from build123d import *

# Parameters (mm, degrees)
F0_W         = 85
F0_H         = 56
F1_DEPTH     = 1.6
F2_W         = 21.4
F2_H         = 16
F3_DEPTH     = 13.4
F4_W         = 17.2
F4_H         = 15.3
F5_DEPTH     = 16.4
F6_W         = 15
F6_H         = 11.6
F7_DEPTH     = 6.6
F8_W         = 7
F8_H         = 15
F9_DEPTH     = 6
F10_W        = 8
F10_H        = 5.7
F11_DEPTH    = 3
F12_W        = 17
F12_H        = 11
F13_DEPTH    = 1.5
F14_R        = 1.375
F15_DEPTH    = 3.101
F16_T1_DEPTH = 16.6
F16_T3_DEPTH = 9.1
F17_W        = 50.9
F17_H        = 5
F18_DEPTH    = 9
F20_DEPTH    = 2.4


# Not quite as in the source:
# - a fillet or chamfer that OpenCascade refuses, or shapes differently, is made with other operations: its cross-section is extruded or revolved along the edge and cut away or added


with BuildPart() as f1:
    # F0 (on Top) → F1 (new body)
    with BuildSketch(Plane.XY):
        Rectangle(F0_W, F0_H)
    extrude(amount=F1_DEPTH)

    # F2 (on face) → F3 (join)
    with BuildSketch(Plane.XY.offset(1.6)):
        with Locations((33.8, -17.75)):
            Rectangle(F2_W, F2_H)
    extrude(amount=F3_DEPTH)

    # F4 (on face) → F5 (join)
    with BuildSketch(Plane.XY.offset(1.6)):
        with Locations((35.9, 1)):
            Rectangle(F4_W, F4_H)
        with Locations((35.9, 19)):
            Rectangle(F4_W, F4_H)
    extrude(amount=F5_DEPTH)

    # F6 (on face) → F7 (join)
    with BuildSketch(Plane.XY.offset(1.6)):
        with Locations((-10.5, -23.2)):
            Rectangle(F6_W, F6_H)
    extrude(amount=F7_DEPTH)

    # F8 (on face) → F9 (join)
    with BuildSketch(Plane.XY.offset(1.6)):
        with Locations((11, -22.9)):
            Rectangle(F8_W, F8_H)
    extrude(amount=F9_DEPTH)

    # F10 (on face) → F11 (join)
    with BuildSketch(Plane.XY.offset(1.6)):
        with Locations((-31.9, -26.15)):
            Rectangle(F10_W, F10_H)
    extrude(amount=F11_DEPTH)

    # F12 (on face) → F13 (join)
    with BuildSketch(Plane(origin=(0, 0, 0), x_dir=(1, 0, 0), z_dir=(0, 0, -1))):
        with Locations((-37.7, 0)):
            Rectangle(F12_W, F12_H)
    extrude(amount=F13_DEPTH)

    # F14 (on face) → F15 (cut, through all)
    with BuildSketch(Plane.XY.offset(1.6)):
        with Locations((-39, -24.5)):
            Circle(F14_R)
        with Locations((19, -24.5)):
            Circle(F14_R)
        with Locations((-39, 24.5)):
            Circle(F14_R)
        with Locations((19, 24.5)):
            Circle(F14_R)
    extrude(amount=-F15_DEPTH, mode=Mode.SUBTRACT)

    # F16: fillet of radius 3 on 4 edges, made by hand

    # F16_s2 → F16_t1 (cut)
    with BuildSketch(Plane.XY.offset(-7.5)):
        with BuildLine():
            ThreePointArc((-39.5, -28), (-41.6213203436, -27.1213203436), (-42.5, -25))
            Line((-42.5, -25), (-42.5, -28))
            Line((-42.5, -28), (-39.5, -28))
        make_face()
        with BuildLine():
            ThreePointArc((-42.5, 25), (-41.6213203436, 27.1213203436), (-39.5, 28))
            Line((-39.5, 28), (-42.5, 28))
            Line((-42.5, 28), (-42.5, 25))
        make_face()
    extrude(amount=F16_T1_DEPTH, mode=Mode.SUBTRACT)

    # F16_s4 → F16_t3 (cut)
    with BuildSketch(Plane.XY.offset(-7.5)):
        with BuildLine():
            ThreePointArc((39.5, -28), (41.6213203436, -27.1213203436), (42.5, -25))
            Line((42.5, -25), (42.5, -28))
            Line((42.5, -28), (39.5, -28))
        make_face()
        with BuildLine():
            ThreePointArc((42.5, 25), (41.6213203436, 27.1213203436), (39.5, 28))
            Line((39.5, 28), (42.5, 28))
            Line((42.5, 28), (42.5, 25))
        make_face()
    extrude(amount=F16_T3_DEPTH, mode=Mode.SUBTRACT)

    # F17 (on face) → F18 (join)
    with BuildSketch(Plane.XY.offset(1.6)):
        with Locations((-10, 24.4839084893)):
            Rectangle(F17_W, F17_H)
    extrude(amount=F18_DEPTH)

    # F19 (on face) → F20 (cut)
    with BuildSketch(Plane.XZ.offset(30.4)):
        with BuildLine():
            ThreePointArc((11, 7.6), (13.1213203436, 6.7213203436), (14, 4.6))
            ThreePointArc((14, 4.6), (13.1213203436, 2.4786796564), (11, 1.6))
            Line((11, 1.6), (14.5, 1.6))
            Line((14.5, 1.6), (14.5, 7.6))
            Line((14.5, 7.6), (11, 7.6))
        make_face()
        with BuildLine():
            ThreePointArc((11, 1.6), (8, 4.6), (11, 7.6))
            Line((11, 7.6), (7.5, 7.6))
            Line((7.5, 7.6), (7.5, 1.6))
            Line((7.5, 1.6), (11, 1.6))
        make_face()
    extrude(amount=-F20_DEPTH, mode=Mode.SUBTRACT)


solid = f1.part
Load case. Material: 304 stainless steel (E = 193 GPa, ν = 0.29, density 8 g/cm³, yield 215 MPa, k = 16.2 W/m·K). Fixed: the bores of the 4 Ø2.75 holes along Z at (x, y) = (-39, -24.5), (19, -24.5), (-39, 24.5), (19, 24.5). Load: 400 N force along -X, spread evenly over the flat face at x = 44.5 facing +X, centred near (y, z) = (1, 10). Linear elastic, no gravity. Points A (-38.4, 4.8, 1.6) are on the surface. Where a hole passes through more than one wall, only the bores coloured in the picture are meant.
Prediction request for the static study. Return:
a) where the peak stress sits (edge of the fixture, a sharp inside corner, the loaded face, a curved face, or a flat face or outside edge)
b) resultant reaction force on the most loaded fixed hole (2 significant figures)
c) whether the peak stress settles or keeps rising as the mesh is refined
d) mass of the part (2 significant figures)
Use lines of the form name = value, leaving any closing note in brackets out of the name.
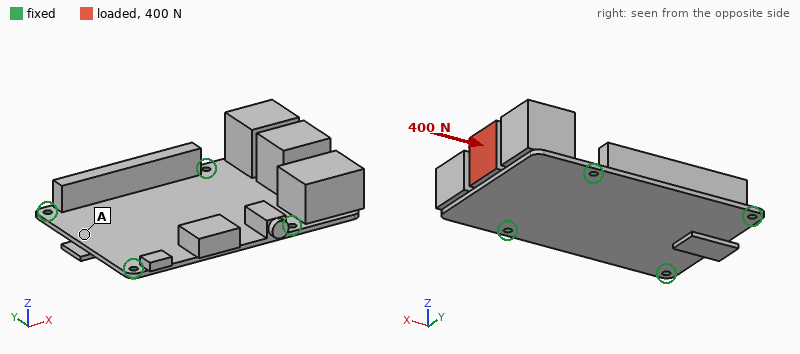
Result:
where the peak stress sits = edge of the fixture
resultant reaction force on the most loaded fixed hole = 150 N
whether the peak stress settles or keeps rising as the mesh is refined = keeps rising
mass of the part = 200 g
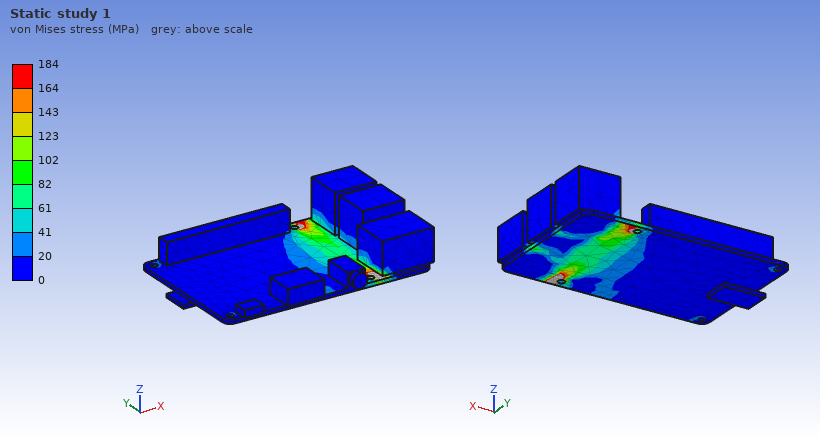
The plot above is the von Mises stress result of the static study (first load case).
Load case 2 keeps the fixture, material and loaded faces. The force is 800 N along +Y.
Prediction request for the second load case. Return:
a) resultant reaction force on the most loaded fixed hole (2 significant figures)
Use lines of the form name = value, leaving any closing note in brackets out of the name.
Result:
resultant reaction force on the most loaded fixed hole = 590 N
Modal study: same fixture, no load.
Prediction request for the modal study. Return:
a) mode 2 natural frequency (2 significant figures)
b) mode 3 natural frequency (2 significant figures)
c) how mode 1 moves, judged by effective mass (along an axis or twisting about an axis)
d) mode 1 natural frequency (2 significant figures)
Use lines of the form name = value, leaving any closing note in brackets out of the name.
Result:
mode 2 natural frequency = 1700 Hz
mode 3 natural frequency = 2000 Hz
how mode 1 moves, judged by effective mass = along Z
mode 1 natural frequency = 530 Hz
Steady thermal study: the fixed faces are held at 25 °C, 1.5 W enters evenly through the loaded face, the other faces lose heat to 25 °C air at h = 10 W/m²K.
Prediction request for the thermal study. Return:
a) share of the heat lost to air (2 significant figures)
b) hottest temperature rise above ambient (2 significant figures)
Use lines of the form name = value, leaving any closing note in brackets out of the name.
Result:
share of the heat lost to air = 51 %
hottest temperature rise above ambient = 20 K
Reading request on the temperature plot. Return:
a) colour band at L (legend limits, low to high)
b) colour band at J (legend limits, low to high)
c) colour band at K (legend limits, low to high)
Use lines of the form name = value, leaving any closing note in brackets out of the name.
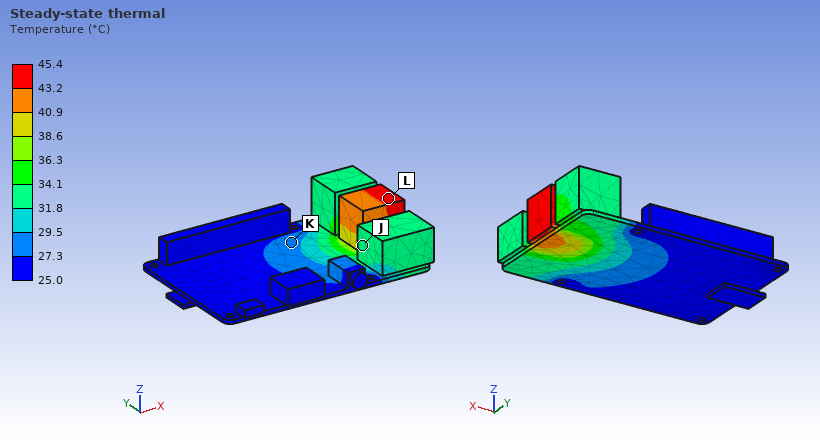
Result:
colour band at L = 43.2 to 45.4 °C
colour band at J = 31.8 to 34.1 °C
colour band at K = 27.3 to 29.5 °C
